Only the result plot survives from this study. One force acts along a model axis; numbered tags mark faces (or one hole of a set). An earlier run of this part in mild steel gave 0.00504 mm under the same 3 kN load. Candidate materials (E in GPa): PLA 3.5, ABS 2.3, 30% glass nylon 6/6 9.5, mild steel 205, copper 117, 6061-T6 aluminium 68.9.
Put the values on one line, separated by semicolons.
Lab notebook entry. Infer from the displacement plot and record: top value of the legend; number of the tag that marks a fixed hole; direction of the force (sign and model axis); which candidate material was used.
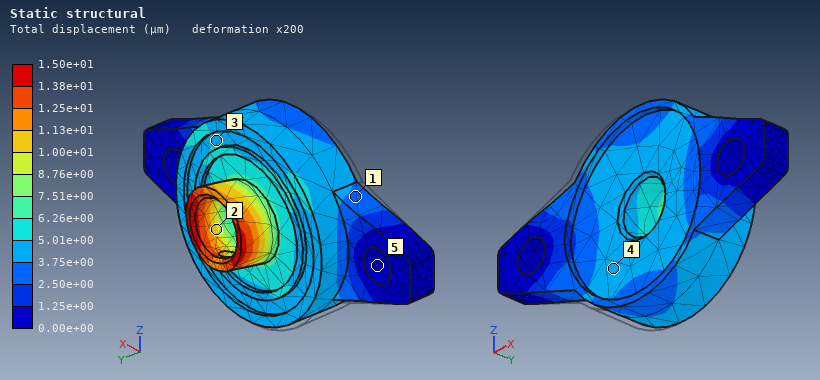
1.50e+01 µm; 5; +X; 6061-T6 aluminium
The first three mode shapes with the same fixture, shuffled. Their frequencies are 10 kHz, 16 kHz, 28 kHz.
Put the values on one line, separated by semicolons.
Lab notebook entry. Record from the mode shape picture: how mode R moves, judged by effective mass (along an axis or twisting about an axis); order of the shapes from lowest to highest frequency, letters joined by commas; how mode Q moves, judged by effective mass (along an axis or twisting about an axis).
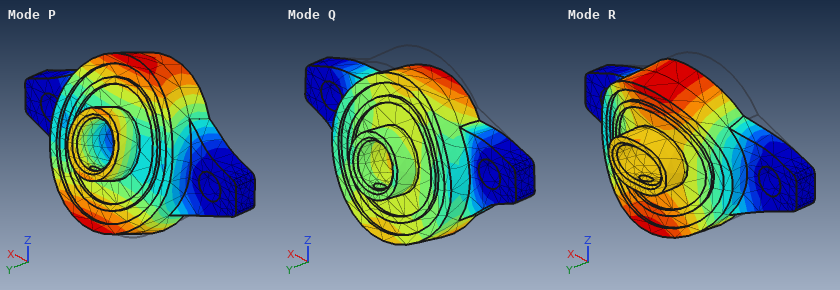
along Y; P, R, Q; along Z
